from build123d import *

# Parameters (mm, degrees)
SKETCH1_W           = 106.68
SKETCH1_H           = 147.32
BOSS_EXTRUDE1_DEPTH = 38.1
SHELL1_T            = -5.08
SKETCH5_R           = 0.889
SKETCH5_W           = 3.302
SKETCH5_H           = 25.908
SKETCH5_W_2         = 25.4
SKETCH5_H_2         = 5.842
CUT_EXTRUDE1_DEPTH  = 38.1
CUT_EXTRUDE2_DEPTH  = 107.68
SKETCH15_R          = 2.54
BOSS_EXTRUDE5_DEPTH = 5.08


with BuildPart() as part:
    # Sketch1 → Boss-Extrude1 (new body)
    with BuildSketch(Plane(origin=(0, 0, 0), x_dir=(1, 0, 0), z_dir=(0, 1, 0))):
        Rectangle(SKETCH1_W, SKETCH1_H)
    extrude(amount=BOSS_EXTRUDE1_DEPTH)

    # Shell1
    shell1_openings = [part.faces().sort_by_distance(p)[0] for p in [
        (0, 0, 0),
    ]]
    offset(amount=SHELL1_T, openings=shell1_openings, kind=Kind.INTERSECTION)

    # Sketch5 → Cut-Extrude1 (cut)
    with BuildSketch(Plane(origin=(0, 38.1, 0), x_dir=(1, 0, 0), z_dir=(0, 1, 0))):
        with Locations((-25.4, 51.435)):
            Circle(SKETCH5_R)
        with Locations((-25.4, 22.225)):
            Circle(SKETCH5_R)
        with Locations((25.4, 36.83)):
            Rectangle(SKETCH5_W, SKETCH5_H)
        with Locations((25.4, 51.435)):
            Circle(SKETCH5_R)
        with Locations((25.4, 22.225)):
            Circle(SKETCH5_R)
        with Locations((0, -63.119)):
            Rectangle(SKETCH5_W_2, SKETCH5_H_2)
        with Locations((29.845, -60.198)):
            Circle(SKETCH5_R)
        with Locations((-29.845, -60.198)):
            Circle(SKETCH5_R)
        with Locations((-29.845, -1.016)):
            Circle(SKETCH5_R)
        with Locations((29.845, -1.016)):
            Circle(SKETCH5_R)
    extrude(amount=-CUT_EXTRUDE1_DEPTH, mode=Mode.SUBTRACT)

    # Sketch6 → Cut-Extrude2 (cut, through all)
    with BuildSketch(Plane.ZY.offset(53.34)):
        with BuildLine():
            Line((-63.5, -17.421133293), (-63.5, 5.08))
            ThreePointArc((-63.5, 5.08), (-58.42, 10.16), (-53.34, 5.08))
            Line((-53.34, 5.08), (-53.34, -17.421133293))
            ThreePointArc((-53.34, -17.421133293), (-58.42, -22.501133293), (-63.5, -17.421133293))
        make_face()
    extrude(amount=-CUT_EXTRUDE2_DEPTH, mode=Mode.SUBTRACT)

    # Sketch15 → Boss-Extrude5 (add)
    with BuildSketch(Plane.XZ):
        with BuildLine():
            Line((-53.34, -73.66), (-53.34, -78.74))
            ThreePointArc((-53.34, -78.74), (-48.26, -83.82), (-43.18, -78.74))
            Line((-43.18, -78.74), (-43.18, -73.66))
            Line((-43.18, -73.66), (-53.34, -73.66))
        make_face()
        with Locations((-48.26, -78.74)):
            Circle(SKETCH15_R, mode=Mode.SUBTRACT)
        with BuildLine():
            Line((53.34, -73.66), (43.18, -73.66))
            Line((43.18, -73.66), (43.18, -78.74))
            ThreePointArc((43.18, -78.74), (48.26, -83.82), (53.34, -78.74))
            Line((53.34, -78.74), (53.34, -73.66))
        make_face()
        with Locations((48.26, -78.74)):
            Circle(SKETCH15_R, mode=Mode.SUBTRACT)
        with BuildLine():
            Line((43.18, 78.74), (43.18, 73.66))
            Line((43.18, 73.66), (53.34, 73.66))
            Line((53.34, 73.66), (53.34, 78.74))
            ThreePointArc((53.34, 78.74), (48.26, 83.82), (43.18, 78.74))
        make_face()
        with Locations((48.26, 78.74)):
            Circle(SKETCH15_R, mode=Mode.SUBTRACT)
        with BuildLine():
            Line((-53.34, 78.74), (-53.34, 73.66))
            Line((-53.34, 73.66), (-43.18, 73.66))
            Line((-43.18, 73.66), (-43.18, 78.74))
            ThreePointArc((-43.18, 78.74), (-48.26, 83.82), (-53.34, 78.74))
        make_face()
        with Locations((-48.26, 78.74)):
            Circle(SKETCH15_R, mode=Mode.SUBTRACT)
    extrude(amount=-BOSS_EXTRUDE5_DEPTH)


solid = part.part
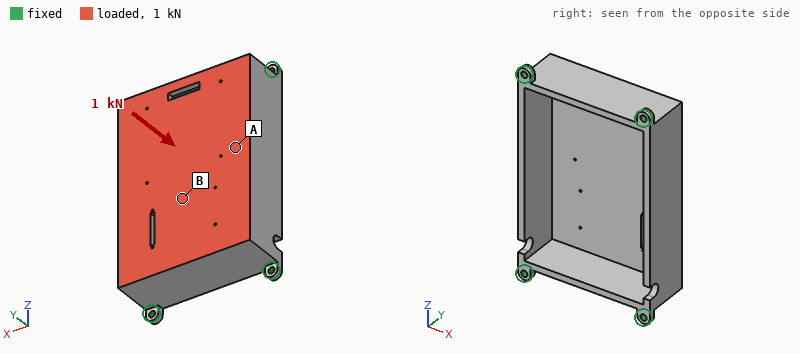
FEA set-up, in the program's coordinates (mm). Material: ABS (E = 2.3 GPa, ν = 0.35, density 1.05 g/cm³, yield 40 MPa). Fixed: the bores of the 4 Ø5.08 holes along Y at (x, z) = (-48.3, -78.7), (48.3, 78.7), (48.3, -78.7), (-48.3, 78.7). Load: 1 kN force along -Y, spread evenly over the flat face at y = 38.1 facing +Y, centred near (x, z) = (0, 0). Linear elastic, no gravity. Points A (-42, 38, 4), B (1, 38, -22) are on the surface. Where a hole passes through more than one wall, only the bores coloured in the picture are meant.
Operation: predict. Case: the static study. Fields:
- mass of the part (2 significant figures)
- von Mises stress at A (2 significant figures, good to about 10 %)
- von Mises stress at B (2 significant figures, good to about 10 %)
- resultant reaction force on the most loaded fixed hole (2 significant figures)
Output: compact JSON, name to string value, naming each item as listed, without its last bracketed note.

{"mass of the part": "170 g", "von Mises stress at A": "2.3 MPa", "von Mises stress at B": "6.6 MPa", "resultant reaction force on the most loaded fixed hole": "310 N"}
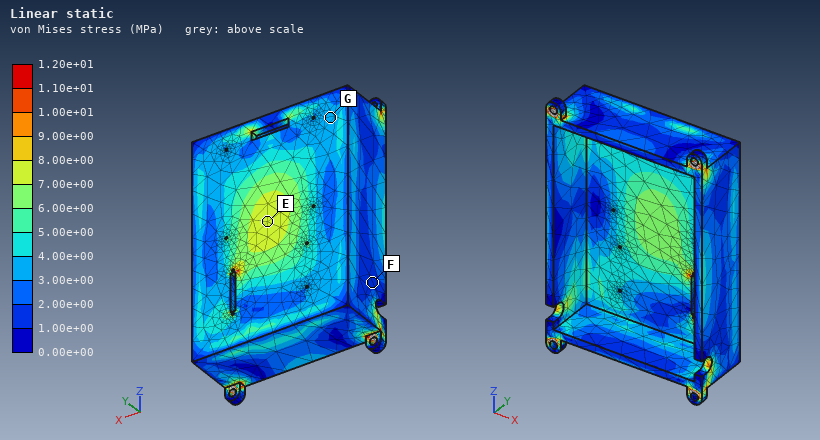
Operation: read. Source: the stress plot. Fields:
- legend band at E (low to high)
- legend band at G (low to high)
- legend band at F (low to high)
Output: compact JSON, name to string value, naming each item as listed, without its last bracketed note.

{"legend band at E": "7.00e+00 to 8.00e+00 MPa", "legend band at G": "3.00e+00 to 4.00e+00 MPa", "legend band at F": "1.00e+00 to 2.00e+00 MPa"}
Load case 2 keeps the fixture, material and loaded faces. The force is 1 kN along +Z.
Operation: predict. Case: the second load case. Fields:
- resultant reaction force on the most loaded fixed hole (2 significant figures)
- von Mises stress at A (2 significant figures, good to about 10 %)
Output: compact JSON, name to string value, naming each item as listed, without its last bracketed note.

{"resultant reaction force on the most loaded fixed hole": "330 N", "von Mises stress at A": "1.2 MPa"}
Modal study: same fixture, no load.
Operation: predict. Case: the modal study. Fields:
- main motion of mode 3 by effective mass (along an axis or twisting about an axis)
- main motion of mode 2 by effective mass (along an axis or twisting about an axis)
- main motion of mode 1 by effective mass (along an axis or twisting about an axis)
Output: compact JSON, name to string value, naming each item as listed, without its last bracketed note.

{"main motion of mode 3 by effective mass": "along Y", "main motion of mode 2 by effective mass": "along X", "main motion of mode 1 by effective mass": "along Y"}
